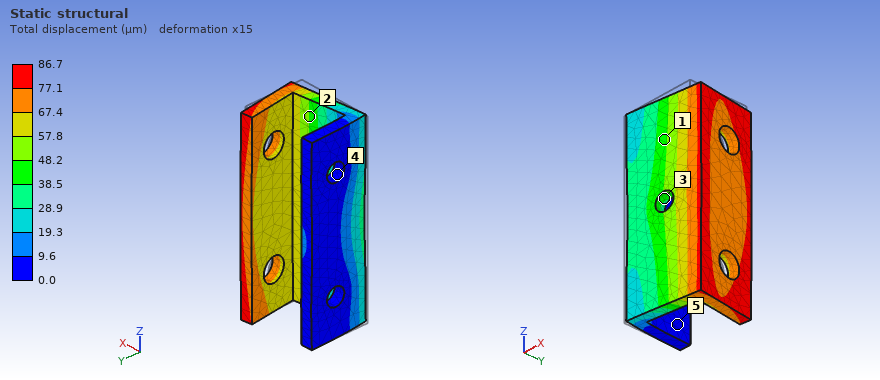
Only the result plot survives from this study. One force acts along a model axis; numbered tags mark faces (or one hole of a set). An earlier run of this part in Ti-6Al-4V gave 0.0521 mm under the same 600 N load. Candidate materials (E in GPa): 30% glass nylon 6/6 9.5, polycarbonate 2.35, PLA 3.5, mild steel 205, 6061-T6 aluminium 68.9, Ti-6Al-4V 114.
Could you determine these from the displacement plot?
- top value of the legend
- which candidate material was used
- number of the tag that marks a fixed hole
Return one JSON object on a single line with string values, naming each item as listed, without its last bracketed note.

{"top value of the legend": "86.7 µm", "which candidate material was used": "6061-T6 aluminium", "number of the tag that marks a fixed hole": "4"}
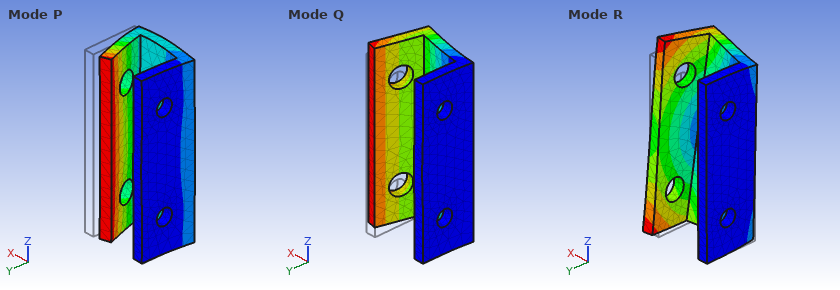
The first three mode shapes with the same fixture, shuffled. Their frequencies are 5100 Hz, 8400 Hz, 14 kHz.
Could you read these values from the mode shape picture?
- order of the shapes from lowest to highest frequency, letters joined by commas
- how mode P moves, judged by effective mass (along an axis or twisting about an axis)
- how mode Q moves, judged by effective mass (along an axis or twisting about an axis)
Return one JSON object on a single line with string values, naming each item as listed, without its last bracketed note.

{"order of the shapes from lowest to highest frequency, letters joined by commas": "Q, R, P", "how mode P moves, judged by effective mass": "along X", "how mode Q moves, judged by effective mass": "along Y"}
